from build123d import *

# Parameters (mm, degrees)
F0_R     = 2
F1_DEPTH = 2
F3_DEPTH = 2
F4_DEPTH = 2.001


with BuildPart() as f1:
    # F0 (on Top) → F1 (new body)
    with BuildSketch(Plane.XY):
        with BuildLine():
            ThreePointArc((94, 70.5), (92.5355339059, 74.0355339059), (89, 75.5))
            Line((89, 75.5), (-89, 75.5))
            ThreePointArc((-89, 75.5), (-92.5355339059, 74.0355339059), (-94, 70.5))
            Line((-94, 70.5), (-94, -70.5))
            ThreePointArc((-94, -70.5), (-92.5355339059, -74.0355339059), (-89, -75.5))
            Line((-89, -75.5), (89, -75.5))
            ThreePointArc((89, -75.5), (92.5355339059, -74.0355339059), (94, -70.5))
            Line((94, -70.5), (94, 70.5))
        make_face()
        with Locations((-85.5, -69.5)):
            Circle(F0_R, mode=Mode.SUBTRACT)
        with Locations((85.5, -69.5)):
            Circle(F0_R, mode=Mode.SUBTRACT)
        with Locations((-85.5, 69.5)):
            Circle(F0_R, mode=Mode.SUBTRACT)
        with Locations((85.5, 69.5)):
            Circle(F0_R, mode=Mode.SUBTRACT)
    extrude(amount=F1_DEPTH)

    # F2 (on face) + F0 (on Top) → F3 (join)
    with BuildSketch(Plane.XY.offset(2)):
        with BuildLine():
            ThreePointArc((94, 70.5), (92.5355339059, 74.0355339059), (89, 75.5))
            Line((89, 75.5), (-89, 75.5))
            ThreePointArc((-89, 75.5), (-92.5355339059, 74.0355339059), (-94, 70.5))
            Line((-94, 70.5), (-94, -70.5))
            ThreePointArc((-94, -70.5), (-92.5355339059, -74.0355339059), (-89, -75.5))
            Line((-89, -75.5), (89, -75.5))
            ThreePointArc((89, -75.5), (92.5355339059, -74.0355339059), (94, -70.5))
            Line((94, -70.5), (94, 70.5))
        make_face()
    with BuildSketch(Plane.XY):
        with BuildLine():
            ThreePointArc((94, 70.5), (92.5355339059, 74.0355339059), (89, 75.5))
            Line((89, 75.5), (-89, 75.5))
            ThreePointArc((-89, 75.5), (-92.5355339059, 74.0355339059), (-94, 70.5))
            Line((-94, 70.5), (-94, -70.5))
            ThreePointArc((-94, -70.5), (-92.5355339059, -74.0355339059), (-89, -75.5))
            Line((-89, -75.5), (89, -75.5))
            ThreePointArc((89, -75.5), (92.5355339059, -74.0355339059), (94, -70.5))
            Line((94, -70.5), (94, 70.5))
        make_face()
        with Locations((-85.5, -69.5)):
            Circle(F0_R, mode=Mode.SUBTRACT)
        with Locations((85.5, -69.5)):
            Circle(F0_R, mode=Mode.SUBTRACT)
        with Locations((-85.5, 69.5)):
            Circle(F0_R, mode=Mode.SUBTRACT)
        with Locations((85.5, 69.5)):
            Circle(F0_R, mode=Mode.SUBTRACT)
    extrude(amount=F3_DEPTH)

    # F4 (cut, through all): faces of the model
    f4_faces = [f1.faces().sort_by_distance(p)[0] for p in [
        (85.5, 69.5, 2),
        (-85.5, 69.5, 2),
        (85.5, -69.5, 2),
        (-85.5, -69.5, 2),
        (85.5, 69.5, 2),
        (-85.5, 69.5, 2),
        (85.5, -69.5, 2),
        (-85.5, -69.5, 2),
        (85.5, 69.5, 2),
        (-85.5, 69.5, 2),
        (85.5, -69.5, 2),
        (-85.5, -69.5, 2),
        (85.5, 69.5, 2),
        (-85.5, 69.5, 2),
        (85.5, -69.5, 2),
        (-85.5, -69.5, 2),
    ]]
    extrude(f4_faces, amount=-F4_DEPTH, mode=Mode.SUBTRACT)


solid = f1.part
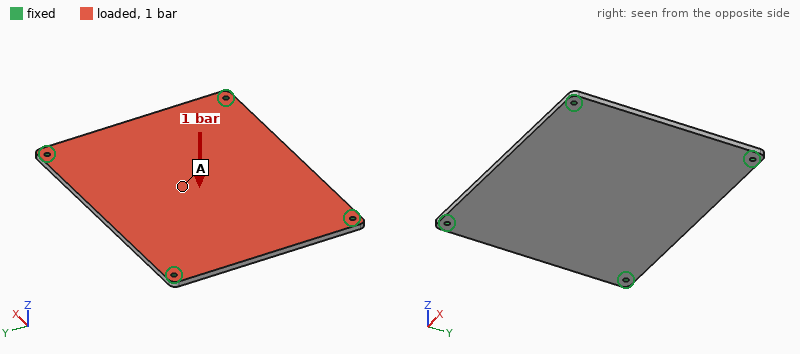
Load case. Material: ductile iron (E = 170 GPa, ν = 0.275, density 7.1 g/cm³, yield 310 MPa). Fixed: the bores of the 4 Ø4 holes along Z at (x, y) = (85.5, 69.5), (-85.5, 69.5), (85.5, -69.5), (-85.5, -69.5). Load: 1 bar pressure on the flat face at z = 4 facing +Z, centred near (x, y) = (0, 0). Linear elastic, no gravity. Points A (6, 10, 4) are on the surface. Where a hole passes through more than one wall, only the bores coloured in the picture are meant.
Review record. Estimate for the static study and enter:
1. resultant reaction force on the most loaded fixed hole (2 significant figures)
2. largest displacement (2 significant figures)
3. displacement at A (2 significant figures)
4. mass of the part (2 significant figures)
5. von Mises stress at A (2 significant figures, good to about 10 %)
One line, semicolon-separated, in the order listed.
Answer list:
710 N; 0.59 mm; 0.59 mm; 800 g; 57 MPa
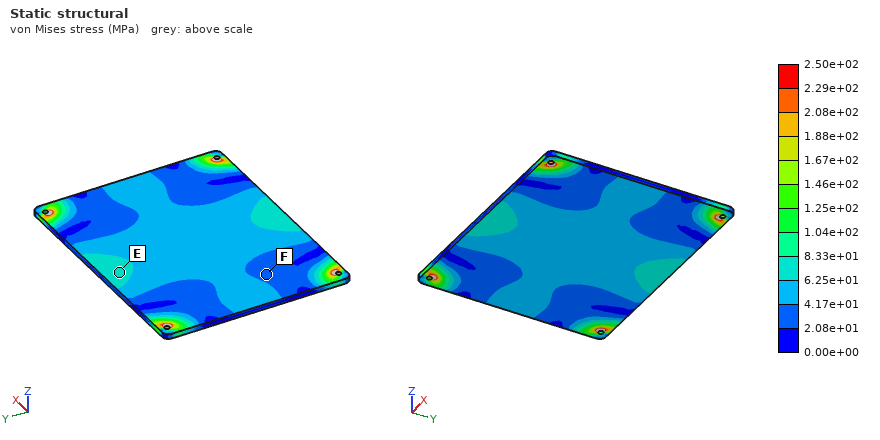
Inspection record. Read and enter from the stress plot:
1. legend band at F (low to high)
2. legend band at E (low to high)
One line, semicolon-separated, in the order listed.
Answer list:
2.08e+01 to 4.17e+01 MPa; 6.25e+01 to 8.33e+01 MPa
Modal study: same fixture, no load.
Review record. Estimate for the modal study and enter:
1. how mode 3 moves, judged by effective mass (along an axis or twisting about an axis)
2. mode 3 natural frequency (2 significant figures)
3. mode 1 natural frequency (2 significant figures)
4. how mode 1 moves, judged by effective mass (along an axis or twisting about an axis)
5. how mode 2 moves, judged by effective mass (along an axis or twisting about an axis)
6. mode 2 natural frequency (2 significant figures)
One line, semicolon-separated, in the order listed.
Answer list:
twisting about Y; 970 Hz; 460 Hz; along Z; twisting about X; 800 Hz
